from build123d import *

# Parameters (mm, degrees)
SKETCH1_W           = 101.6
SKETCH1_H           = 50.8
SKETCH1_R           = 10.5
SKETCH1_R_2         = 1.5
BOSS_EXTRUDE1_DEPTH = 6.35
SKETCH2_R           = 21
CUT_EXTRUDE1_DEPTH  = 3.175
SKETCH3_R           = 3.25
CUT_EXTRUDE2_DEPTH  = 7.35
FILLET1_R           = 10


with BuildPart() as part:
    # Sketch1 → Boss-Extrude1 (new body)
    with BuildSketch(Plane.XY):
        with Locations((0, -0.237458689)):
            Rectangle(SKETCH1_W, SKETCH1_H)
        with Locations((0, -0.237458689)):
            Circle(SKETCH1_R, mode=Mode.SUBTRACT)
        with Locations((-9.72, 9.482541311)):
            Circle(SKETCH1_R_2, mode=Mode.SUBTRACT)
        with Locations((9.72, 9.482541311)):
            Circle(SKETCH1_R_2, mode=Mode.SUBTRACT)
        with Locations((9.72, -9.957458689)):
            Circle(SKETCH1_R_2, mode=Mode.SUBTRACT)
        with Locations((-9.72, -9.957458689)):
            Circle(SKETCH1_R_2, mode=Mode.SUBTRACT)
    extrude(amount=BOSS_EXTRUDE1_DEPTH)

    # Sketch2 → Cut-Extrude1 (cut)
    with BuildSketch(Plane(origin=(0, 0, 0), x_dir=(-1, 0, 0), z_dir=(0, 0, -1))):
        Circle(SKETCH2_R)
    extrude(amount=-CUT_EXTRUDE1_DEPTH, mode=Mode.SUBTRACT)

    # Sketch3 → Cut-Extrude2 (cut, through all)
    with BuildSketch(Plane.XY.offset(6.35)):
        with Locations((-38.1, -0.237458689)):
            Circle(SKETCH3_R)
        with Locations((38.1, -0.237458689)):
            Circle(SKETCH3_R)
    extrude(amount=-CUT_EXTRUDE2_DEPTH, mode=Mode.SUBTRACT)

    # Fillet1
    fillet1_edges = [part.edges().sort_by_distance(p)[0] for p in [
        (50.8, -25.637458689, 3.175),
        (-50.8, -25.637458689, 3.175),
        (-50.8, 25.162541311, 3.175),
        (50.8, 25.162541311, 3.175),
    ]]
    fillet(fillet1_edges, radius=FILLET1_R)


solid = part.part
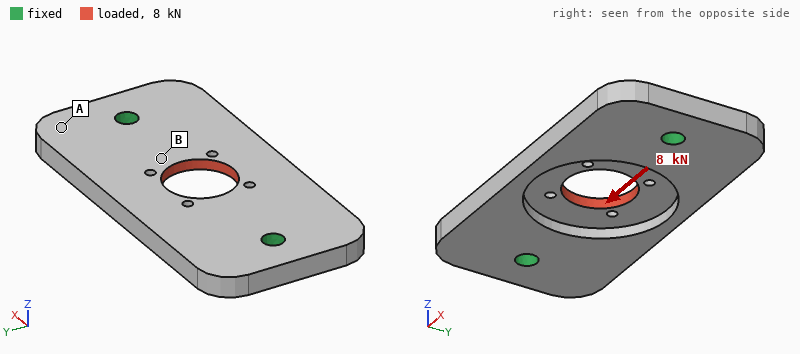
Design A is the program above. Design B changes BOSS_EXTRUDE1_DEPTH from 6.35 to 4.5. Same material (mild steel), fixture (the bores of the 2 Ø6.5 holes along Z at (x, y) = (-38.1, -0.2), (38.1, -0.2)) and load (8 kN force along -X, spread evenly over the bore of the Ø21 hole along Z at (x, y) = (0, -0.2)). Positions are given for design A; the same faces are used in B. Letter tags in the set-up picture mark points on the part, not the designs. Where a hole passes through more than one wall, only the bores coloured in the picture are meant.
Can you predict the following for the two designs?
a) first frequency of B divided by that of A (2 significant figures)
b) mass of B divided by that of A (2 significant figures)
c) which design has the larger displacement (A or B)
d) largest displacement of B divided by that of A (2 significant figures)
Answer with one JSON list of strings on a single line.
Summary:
["0.76", "0.67", "B", "2.4"]
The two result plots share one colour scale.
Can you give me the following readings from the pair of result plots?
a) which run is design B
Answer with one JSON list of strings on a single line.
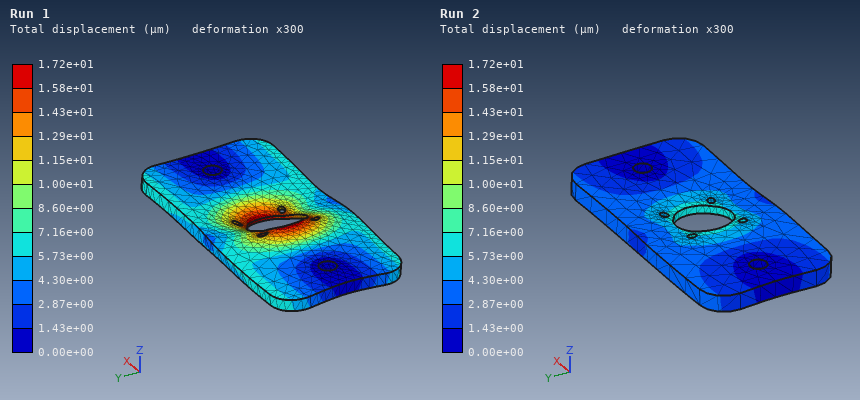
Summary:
["Run 1"]
